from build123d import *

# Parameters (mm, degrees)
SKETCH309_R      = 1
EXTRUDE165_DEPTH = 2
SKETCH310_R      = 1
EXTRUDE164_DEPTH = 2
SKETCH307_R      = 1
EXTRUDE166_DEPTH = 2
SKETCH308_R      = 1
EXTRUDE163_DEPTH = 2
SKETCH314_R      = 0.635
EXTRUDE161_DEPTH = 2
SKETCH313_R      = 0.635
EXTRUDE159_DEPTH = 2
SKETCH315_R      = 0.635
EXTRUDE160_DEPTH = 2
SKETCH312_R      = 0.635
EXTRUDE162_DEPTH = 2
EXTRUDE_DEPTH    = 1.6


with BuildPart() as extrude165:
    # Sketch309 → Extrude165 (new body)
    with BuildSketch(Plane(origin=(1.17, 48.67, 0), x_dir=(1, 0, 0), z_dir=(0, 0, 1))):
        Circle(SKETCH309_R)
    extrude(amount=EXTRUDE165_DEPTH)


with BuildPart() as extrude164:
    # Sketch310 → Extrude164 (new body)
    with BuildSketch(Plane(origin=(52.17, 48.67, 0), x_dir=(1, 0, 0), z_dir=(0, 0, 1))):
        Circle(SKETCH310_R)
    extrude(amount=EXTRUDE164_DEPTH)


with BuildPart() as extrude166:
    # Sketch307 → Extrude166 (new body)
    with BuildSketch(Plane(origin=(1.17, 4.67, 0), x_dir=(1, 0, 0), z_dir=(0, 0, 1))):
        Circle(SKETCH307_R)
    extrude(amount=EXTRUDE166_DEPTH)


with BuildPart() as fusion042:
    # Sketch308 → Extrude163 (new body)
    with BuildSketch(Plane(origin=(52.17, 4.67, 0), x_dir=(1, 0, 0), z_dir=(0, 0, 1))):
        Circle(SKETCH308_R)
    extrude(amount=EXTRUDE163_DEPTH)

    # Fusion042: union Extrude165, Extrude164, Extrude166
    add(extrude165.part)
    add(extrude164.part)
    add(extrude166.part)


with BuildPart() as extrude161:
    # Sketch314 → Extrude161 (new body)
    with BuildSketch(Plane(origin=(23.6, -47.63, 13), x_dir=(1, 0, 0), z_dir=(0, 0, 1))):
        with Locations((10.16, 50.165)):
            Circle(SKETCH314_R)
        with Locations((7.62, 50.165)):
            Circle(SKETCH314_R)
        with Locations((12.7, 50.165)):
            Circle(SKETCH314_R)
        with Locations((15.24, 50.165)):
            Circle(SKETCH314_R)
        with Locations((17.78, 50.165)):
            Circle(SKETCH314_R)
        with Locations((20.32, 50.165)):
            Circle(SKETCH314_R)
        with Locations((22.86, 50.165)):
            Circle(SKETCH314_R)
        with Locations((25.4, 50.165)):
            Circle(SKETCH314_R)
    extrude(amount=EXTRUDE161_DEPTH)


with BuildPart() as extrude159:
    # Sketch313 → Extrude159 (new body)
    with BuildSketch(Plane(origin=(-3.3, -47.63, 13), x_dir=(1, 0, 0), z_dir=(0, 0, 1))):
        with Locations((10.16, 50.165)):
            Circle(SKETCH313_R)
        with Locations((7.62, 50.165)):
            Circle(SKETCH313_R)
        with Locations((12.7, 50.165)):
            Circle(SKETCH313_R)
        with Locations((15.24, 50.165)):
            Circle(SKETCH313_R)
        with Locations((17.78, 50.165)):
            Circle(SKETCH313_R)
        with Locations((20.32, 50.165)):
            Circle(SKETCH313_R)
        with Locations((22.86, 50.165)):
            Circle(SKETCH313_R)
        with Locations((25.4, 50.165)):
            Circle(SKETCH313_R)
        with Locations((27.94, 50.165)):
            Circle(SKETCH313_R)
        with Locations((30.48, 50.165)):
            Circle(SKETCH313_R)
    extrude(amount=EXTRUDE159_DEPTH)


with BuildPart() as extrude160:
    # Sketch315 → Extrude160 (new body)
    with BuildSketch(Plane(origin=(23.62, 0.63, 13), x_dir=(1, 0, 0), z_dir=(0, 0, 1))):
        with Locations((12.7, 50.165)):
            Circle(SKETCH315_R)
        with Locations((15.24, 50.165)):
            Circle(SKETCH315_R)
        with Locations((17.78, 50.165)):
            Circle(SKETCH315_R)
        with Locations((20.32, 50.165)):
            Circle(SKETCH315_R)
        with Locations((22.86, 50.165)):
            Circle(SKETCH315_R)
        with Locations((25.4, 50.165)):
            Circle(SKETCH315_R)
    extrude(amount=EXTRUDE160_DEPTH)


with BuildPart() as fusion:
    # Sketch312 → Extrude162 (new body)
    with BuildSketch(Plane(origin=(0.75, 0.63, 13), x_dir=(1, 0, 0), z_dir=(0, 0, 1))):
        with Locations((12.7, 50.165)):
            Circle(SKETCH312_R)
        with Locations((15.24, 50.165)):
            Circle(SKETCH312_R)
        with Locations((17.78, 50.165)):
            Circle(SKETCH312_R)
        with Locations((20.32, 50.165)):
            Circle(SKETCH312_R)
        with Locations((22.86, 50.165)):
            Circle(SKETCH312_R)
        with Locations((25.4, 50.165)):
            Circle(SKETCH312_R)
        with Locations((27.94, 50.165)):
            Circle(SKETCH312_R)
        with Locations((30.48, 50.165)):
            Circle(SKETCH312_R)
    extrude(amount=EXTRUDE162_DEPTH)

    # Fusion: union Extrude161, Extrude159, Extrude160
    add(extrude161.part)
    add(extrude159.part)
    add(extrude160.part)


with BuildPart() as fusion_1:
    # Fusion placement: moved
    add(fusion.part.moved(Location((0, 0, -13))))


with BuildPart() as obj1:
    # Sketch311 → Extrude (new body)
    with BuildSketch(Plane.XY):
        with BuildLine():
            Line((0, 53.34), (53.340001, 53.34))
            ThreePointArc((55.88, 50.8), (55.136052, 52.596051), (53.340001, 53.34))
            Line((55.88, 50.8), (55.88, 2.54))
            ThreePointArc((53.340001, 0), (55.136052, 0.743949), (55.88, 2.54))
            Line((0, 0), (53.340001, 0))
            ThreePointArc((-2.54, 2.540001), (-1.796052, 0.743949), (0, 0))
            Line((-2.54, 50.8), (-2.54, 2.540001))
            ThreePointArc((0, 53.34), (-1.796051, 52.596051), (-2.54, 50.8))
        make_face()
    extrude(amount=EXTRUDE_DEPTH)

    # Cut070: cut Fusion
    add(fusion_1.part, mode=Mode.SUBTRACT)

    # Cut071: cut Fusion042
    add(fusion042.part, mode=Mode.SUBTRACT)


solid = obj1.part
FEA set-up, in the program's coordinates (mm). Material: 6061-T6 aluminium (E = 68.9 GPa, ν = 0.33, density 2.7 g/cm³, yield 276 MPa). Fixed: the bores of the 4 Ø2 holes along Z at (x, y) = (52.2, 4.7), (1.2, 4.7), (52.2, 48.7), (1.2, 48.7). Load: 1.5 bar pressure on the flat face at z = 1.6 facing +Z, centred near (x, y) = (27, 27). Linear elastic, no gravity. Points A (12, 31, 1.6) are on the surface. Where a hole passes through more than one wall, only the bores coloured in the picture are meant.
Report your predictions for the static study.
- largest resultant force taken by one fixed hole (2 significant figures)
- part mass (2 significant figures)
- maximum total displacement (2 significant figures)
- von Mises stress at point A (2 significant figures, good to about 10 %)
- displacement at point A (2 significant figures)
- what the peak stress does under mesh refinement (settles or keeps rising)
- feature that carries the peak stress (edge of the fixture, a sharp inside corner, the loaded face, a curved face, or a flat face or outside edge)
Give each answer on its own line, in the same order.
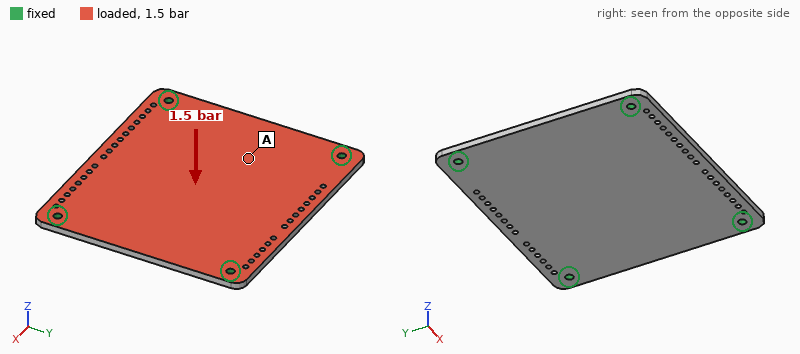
120 N
13 g
0.24 mm
34 MPa
0.17 mm
keeps rising
edge of the fixture
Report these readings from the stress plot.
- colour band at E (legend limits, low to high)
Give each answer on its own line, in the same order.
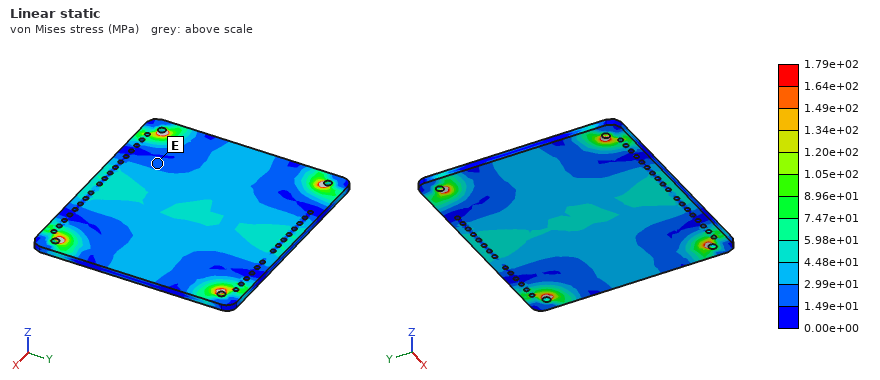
1.49e+01 to 2.99e+01 MPa
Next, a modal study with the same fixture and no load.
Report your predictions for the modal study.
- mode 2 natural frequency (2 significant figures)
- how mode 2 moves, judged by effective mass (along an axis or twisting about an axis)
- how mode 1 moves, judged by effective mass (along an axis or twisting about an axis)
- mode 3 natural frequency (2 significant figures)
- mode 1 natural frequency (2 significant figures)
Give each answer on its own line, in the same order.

3600 Hz
twisting about X
along Z
4400 Hz
2300 Hz
